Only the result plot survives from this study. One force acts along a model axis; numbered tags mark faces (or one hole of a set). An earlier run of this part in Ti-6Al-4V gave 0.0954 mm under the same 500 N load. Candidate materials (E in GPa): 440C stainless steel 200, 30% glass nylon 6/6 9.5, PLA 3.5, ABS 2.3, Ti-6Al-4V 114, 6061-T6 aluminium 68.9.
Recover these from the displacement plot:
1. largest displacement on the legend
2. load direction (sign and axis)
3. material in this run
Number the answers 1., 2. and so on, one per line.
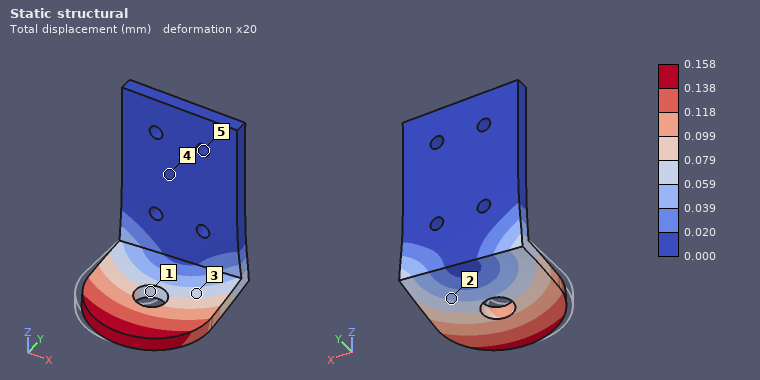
1. 0.158 mm
2. +X
3. 6061-T6 aluminium
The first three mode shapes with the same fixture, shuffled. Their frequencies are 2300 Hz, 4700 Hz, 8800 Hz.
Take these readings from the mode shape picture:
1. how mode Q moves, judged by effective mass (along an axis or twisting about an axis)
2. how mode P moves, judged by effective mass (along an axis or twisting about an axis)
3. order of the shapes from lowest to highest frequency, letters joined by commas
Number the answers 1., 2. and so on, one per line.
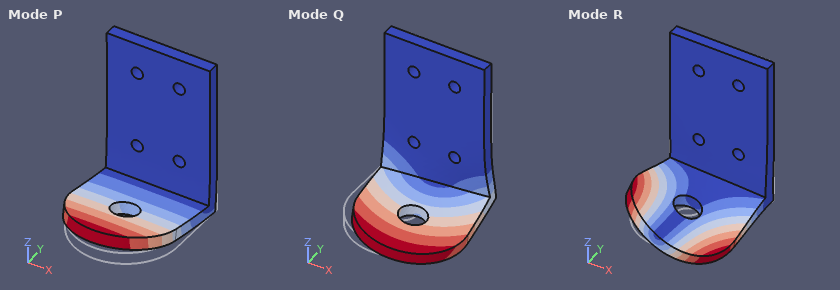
1. along X
2. along Z
3. P, Q, R
